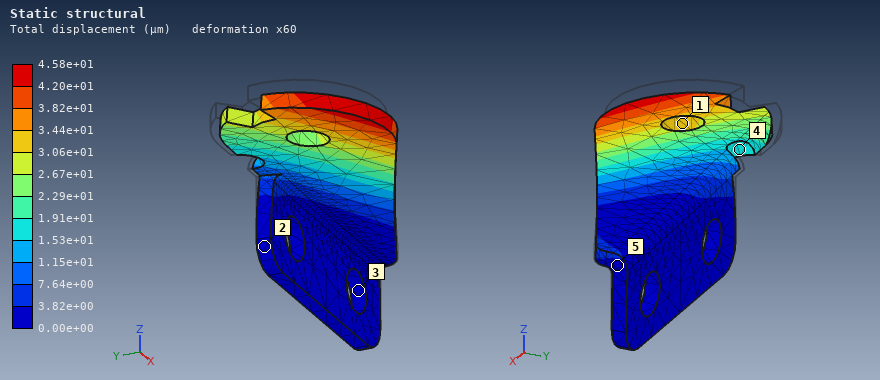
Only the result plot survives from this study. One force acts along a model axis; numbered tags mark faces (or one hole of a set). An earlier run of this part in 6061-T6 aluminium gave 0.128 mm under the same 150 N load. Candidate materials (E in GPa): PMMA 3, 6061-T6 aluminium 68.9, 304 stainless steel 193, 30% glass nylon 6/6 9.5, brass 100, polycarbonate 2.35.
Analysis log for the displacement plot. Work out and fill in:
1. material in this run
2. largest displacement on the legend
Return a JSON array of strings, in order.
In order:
["304 stainless steel", "4.58e+01 µm"]
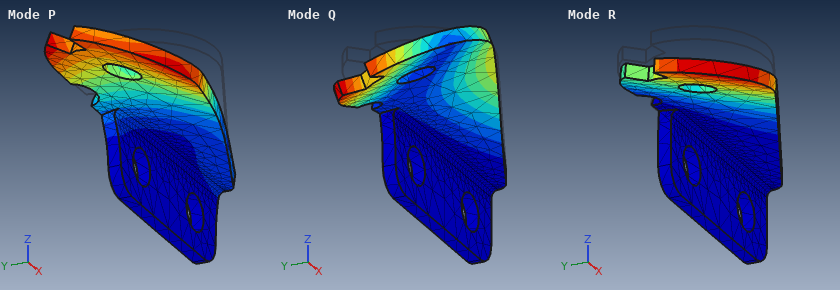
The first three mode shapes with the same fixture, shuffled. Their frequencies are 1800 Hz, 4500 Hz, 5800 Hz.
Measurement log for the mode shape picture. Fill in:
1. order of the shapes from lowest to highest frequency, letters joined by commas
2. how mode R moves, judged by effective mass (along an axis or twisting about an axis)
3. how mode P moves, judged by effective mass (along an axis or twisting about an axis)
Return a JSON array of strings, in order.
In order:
["R, Q, P", "along Z", "along Y"]
